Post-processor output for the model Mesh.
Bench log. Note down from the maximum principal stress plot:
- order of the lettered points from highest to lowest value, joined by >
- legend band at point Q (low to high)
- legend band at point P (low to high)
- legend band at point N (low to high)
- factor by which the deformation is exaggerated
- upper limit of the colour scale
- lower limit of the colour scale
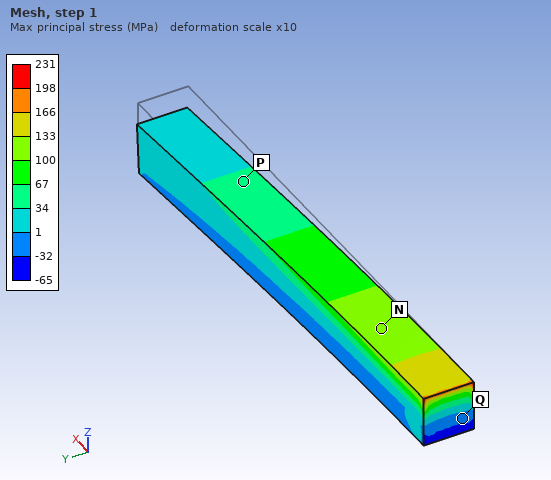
N > P > Q
-32 to 1 MPa
34 to 67 MPa
100 to 133 MPa
10
231 MPa
-65 MPa
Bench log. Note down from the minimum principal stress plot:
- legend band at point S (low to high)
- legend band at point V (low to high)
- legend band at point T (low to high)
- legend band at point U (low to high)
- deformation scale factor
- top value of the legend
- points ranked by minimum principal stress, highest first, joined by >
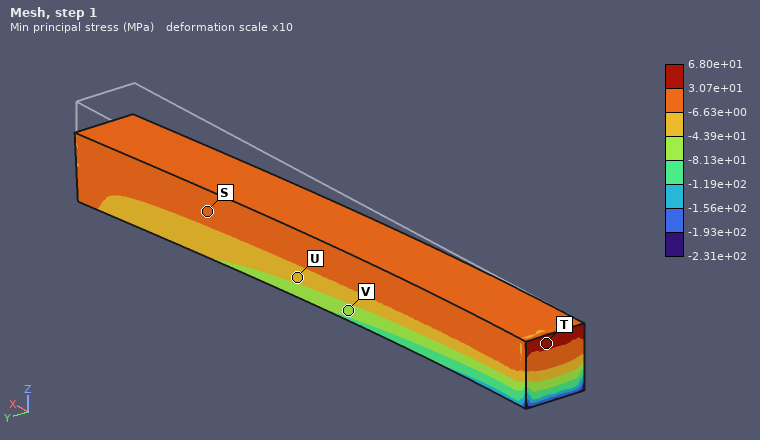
-6.63e+00 to 3.07e+01 MPa
-8.13e+01 to -4.39e+01 MPa
3.07e+01 to 6.80e+01 MPa
-4.39e+01 to -6.63e+00 MPa
10
6.80e+01 MPa
T > S > U > V
